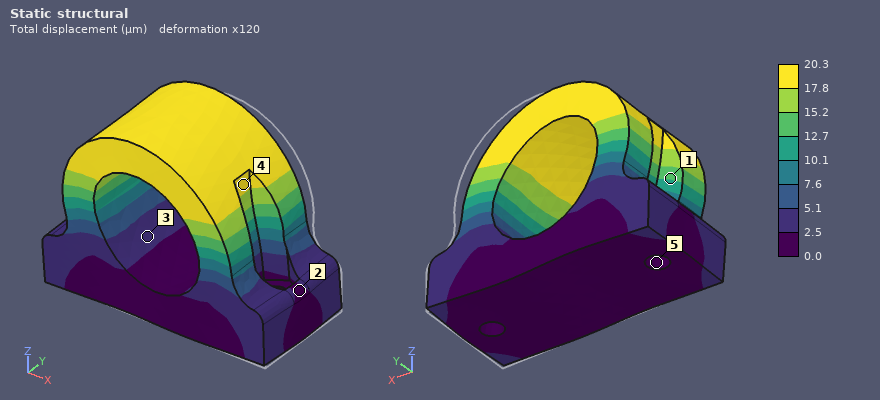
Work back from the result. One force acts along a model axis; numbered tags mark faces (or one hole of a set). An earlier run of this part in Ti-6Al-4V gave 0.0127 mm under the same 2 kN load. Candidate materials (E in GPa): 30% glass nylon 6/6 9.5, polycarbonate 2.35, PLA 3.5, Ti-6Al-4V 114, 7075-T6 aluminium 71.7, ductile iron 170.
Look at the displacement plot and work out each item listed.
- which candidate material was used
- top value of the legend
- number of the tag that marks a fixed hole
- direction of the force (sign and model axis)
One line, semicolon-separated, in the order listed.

7075-T6 aluminium; 20.3 µm; 5; -X
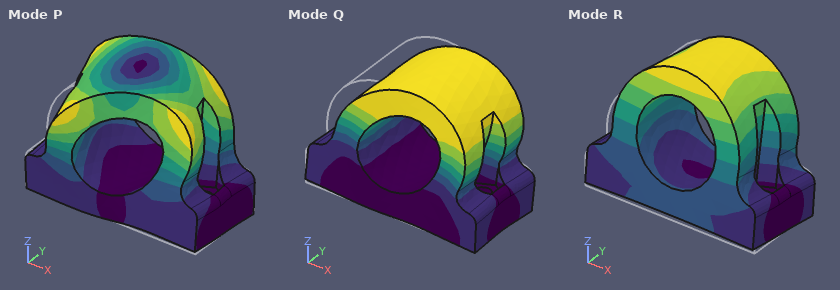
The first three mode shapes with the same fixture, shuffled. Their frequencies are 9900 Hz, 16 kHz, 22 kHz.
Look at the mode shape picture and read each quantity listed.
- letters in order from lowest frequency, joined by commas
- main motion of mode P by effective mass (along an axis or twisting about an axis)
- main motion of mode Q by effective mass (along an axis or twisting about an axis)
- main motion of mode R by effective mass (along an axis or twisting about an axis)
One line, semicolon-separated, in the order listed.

R, Q, P; twisting about Z; along X; along Y
